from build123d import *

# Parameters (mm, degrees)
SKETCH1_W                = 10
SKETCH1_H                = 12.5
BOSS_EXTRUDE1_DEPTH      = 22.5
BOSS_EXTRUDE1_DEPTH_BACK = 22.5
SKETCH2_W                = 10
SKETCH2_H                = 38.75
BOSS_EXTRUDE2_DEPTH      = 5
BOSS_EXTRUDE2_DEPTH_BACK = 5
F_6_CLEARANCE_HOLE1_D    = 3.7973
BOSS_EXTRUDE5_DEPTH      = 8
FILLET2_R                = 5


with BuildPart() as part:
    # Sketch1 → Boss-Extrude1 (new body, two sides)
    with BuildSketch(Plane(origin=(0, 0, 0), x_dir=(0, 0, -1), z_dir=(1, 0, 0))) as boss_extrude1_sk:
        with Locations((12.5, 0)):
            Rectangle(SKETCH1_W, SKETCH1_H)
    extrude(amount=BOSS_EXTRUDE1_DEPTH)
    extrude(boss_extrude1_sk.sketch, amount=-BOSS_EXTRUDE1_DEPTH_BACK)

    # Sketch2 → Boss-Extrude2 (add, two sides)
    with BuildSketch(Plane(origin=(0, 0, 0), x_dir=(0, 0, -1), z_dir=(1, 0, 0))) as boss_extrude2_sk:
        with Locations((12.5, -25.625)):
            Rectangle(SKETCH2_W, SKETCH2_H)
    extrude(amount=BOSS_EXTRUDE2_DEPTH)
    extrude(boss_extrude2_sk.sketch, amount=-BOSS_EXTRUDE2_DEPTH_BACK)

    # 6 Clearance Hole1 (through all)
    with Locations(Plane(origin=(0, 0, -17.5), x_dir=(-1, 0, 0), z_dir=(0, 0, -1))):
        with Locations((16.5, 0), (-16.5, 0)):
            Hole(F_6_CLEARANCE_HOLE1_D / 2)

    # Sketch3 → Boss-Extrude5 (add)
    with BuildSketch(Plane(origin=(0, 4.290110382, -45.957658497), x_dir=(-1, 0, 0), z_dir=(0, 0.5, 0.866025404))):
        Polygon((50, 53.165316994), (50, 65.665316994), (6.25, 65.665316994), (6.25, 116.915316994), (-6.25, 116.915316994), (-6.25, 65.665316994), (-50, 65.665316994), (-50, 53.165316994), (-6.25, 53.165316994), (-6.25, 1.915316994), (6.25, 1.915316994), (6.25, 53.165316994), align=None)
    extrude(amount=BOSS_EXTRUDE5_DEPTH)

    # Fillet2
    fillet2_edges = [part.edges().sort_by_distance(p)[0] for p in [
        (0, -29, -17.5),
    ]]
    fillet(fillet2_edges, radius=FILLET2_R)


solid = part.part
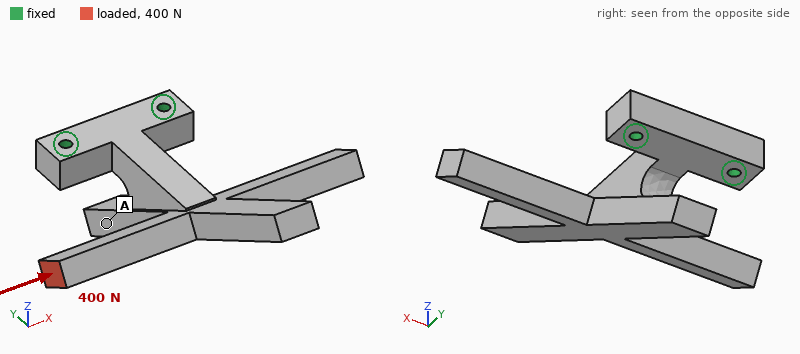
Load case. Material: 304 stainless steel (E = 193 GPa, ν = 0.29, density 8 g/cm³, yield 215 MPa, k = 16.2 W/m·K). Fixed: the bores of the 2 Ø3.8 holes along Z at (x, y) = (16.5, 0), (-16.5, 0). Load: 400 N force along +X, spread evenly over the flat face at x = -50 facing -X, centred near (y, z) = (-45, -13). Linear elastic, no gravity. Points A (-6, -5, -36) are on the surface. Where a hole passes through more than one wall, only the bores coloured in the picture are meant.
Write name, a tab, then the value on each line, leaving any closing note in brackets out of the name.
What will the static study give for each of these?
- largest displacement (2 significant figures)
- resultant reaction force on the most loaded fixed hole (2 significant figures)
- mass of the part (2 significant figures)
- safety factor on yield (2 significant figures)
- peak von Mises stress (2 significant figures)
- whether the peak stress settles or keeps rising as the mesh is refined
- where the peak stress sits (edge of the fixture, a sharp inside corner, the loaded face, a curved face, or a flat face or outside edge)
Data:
largest displacement	0.16 mm
resultant reaction force on the most loaded fixed hole	670 N
mass of the part	240 g
safety factor on yield	2.1
peak von Mises stress	100 MPa
whether the peak stress settles or keeps rising as the mesh is refined	settles
where the peak stress sits	a curved face
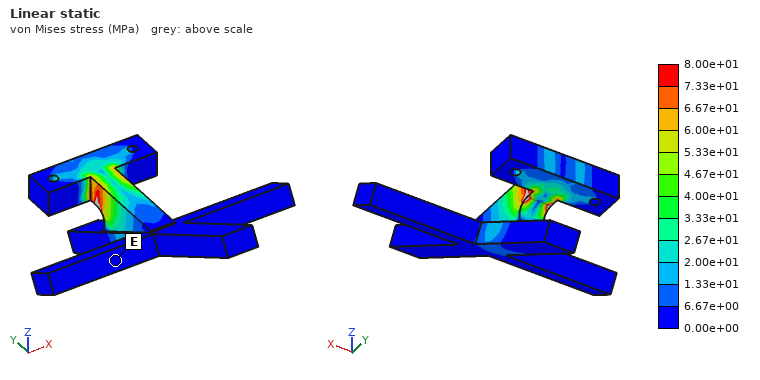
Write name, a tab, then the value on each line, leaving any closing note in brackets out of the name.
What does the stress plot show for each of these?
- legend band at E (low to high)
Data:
legend band at E	0.00e+00 to 6.67e+00 MPa
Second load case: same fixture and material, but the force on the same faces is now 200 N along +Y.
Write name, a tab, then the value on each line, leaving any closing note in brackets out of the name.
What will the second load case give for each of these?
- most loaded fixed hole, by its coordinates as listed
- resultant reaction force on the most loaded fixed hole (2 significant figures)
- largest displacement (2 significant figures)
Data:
most loaded fixed hole, by its coordinates as listed	(-16.5, 0)
resultant reaction force on the most loaded fixed hole	460 N
largest displacement	0.15 mm
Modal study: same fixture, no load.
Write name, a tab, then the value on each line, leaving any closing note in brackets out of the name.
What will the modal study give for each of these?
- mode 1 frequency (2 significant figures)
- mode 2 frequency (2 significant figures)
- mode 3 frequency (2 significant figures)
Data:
mode 1 frequency	690 Hz
mode 2 frequency	710 Hz
mode 3 frequency	1200 Hz
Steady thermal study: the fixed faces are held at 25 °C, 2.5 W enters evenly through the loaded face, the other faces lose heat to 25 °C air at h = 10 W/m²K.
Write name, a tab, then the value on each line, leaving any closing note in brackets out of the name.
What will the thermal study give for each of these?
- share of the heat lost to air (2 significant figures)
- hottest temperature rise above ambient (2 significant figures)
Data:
share of the heat lost to air	71 %
hottest temperature rise above ambient	75 K
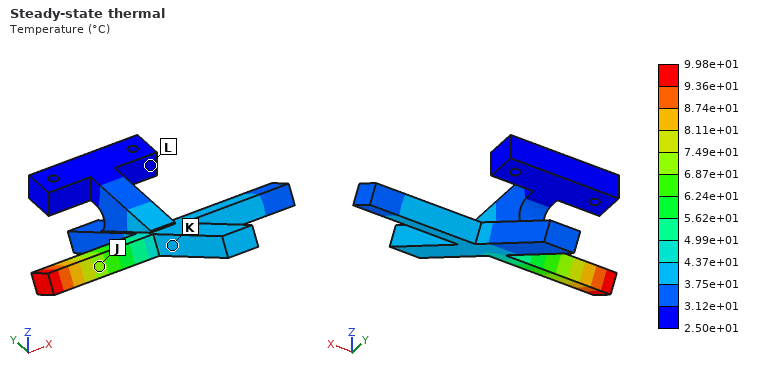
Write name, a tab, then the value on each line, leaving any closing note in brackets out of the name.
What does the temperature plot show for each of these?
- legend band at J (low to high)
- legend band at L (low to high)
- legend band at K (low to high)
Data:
legend band at J	6.87e+01 to 7.49e+01 °C
legend band at L	2.50e+01 to 3.12e+01 °C
legend band at K	3.75e+01 to 4.37e+01 °C
